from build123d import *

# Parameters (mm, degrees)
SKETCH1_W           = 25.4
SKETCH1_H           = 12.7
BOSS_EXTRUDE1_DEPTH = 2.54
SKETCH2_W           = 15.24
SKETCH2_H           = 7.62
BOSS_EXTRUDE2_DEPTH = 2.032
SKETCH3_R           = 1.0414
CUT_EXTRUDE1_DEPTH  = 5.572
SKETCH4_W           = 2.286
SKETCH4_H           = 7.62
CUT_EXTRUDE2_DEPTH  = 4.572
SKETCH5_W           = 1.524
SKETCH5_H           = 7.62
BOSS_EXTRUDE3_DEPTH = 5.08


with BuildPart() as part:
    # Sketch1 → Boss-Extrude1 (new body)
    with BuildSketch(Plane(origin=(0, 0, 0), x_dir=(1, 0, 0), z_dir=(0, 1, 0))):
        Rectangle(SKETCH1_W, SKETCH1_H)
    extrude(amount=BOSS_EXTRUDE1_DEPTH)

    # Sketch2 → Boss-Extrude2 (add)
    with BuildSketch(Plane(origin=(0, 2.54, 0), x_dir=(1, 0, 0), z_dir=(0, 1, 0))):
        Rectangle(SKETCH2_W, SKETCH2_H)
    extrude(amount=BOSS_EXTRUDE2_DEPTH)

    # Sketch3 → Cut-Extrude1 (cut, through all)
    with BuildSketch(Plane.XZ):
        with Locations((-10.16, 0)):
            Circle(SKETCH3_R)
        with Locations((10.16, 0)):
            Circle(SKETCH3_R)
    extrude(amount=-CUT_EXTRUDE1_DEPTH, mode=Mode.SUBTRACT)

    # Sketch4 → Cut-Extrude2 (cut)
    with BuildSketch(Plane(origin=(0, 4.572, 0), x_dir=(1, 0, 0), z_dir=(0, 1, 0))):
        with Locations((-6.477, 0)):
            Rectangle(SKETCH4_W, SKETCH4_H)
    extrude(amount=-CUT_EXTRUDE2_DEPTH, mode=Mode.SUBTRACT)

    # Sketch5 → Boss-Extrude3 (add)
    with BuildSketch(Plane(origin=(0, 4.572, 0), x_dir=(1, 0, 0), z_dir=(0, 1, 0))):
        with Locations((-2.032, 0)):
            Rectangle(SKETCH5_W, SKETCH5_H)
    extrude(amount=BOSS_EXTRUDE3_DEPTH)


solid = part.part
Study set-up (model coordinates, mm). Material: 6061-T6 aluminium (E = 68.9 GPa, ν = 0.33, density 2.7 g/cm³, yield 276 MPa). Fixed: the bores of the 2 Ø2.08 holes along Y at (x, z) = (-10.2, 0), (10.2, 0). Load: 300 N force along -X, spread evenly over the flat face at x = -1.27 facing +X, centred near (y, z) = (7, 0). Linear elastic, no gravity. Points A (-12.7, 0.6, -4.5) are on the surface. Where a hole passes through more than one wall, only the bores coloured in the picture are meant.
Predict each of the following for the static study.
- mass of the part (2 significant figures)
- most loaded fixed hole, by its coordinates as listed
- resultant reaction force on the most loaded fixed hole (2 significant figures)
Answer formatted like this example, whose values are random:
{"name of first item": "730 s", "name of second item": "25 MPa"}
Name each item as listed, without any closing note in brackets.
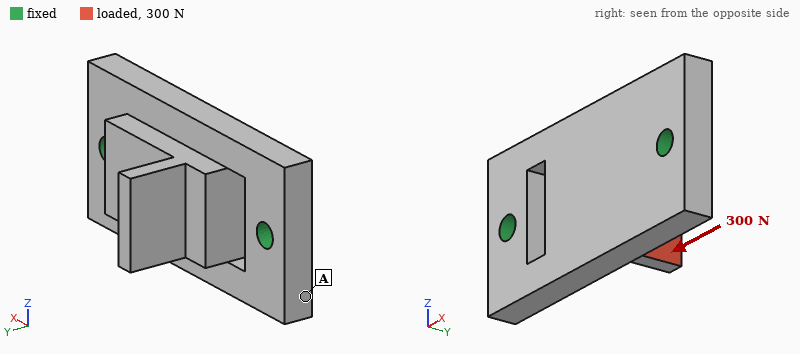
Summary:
{"mass of the part": "2.7 g", "most loaded fixed hole, by its coordinates as listed": "(10.2, 0)", "resultant reaction force on the most loaded fixed hole": "280 N"}
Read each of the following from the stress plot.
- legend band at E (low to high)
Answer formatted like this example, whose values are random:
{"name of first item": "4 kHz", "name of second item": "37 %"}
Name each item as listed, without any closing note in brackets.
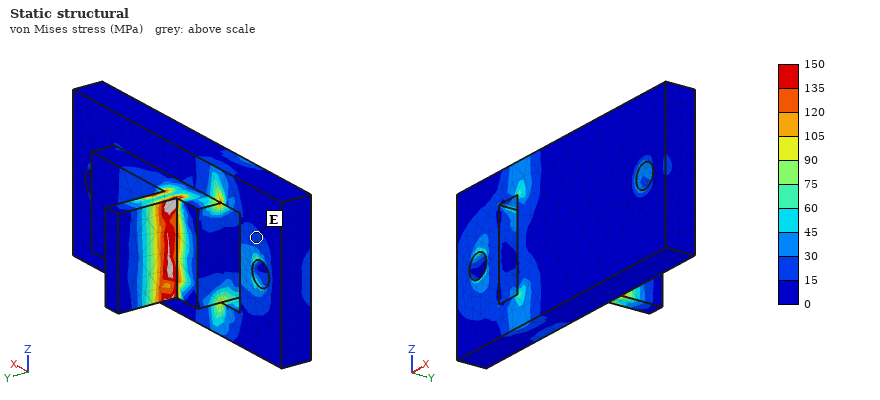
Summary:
{"legend band at E": "15 to 30 MPa"}
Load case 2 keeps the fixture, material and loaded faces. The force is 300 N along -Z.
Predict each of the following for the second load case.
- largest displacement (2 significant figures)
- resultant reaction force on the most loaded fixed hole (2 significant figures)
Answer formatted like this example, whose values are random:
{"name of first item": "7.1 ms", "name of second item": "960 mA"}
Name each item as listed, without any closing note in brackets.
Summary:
{"largest displacement": "47 µm", "resultant reaction force on the most loaded fixed hole": "150 N"}
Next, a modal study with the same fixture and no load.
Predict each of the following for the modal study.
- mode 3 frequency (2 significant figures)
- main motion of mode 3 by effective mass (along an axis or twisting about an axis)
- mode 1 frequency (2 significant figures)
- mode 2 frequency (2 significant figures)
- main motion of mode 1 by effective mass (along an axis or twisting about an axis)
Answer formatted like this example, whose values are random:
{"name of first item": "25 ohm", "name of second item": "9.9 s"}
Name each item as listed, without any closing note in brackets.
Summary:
{"mode 3 frequency": "33 kHz", "main motion of mode 3 by effective mass": "along Z", "mode 1 frequency": "19 kHz", "mode 2 frequency": "21 kHz", "main motion of mode 1 by effective mass": "along Y"}
